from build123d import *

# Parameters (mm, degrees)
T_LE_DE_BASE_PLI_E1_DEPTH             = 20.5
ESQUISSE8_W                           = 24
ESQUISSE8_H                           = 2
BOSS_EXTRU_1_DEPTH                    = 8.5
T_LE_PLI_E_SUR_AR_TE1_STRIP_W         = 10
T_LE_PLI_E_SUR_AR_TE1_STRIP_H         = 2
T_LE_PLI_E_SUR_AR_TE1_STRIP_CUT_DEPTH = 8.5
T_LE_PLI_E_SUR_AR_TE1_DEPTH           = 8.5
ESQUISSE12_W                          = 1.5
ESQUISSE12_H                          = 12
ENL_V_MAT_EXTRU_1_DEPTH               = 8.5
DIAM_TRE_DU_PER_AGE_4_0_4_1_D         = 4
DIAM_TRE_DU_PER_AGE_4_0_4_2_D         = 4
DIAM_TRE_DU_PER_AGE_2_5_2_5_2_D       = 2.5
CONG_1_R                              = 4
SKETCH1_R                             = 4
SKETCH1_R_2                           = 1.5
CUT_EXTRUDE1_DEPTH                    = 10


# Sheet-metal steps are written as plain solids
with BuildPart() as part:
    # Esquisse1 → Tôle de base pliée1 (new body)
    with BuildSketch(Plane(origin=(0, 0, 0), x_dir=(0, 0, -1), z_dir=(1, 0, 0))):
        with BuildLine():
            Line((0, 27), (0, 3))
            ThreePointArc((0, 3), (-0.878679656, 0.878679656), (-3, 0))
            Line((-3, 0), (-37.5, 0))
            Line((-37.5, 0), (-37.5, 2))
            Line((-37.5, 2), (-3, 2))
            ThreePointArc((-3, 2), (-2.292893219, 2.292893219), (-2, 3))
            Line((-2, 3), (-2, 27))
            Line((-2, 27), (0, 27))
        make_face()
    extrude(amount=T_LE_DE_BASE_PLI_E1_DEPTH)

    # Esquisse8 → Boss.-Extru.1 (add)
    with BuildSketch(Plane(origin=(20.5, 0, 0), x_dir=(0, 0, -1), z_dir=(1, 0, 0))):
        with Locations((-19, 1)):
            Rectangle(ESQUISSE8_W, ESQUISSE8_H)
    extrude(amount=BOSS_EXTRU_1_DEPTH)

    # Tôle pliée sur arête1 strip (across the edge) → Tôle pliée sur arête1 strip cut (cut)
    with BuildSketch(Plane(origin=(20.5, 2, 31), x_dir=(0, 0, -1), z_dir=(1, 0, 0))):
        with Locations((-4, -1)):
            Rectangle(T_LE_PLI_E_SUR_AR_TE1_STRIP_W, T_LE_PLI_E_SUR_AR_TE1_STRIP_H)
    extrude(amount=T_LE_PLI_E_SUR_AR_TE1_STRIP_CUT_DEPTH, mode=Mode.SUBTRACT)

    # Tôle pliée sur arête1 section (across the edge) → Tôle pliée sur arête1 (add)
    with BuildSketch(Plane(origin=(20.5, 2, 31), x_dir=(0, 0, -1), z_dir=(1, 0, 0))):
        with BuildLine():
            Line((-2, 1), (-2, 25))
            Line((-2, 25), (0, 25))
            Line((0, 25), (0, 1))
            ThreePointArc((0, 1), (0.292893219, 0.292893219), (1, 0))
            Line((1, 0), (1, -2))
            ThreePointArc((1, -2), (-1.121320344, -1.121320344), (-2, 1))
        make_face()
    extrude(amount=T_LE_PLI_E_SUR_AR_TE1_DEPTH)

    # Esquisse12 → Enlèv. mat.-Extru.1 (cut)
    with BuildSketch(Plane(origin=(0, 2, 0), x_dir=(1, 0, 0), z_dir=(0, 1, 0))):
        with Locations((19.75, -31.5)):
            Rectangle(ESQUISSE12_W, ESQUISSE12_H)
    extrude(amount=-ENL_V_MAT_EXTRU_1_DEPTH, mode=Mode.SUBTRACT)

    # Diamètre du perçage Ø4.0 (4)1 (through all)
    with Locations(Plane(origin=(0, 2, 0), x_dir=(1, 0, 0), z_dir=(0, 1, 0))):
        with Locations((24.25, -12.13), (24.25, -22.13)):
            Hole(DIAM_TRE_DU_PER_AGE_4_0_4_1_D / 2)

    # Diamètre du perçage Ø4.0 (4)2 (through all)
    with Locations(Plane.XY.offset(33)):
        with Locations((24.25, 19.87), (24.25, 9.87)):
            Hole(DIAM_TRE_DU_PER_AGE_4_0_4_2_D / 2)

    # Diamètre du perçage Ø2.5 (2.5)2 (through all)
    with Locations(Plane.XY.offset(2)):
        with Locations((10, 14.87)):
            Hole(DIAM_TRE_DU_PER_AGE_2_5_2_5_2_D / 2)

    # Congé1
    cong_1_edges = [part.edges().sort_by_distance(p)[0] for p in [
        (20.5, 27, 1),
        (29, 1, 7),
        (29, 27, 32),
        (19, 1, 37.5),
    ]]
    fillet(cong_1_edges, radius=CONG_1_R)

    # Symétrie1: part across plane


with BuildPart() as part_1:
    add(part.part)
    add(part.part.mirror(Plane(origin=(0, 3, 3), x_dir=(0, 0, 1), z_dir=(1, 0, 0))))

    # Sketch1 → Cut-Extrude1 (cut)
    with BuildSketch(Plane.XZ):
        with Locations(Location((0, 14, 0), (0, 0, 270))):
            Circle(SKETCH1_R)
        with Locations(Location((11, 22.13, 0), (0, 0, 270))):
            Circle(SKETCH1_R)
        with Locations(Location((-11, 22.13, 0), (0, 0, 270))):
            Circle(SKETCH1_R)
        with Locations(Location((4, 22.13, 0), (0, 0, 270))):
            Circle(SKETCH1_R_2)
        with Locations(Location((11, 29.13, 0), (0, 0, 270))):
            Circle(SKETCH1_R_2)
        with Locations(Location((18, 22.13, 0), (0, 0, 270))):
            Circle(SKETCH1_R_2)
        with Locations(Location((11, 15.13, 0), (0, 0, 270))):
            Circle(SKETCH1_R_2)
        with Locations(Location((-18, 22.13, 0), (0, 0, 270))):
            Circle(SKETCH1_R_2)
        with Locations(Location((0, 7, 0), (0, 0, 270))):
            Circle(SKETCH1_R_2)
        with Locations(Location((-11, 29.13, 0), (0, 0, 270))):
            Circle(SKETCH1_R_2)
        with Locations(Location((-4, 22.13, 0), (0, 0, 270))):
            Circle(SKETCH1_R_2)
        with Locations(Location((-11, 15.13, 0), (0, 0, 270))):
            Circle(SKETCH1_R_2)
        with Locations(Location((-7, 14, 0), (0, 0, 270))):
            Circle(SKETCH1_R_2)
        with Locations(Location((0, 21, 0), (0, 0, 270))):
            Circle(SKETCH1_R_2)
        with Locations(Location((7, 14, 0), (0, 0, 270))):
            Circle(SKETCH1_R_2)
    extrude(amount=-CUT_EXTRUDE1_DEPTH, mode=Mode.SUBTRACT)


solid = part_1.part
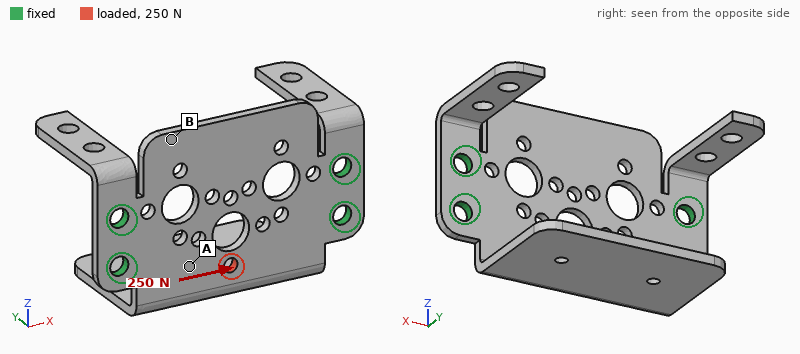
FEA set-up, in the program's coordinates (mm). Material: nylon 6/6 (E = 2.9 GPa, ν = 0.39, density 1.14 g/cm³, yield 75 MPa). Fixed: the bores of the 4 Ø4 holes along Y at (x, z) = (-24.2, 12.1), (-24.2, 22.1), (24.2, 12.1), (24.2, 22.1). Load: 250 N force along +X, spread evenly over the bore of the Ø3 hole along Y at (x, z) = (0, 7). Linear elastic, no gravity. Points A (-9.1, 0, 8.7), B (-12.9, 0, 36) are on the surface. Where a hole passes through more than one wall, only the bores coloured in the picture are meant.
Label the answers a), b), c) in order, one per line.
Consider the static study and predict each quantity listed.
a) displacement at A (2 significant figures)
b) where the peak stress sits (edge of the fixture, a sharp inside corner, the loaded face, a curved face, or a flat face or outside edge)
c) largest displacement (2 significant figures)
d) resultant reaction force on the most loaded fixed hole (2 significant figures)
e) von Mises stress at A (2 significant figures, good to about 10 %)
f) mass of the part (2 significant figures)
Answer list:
a) 34 µm
b) a sharp inside corner
c) 61 µm
d) 110 N
e) 7.0 MPa
f) 6.8 g
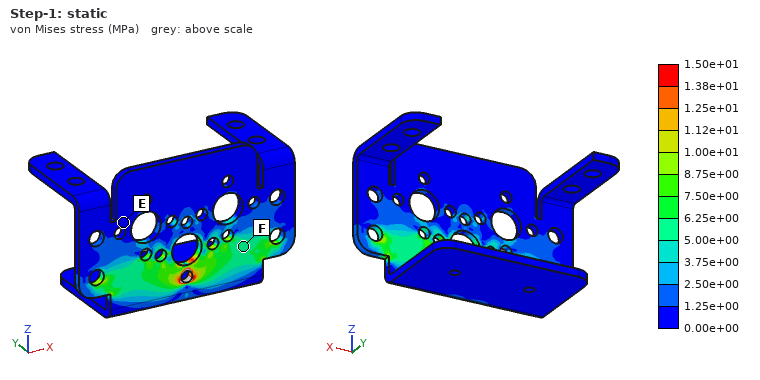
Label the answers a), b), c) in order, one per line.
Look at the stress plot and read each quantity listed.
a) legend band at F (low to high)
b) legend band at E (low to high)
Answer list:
a) 5.00e+00 to 6.25e+00 MPa
b) 0.00e+00 to 1.25e+00 MPa
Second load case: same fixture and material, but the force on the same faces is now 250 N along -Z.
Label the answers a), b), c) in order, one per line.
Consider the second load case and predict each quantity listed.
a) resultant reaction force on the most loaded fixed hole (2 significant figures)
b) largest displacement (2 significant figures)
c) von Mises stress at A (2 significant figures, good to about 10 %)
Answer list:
a) 89 N
b) 0.15 mm
c) 5.7 MPa
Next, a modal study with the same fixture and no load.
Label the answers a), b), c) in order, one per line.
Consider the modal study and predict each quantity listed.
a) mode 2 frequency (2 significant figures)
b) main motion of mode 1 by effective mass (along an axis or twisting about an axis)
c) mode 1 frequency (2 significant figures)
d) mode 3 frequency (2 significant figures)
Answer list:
a) 550 Hz
b) along Z
c) 420 Hz
d) 550 Hz
